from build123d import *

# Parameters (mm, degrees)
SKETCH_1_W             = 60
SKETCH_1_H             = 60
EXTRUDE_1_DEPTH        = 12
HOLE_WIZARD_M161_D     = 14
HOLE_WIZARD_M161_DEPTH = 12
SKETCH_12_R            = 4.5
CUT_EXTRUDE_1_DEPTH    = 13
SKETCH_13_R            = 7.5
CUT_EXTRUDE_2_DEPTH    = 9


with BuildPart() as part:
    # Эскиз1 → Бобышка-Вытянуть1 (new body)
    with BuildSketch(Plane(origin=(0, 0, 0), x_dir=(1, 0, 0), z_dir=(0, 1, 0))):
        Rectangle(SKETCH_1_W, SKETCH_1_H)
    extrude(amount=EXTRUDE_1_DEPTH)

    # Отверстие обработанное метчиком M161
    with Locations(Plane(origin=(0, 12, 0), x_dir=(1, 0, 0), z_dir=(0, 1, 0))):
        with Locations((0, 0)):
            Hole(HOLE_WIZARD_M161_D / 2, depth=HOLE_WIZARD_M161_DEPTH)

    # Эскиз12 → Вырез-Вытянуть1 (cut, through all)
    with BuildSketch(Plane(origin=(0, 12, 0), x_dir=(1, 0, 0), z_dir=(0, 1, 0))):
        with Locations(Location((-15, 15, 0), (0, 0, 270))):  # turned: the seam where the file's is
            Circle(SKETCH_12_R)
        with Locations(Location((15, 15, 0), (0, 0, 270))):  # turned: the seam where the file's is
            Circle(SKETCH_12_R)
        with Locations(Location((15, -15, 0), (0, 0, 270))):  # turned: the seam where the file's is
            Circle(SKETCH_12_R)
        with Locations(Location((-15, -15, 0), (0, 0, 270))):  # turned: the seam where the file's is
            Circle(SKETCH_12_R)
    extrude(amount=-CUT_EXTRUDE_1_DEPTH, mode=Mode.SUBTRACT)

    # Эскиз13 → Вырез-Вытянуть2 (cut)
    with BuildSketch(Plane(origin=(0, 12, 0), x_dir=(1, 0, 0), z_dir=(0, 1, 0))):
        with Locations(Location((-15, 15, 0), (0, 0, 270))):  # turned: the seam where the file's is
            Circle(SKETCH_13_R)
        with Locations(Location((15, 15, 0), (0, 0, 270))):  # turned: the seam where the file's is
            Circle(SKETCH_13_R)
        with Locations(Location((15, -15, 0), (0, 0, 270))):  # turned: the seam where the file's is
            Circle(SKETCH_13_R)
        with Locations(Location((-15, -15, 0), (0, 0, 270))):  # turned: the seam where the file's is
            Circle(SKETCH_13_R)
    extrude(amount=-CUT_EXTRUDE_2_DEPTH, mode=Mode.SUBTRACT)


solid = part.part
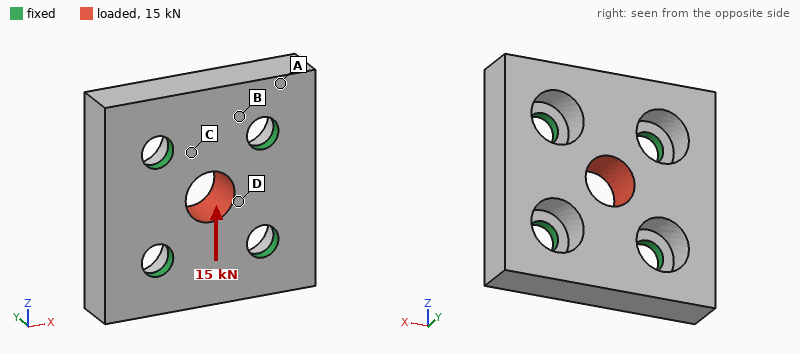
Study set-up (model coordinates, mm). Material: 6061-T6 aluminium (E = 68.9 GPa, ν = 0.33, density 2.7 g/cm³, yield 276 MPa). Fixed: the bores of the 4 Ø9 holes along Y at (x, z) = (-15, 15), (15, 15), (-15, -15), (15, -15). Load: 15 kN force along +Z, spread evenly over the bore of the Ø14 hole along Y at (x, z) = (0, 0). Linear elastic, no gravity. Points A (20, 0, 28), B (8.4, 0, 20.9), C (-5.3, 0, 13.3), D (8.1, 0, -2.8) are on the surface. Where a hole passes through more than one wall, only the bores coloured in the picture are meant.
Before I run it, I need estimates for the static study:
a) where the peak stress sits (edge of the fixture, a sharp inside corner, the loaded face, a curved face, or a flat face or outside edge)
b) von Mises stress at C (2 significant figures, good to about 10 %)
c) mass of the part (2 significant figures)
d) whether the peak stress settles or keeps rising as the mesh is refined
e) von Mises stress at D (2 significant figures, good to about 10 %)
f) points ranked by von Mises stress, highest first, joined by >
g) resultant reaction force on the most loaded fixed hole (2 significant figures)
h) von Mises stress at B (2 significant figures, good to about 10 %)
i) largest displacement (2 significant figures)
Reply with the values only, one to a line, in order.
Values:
edge of the fixture
20 MPa
92 g
keeps rising
52 MPa
D > B > C > A
4.0 kN
40 MPa
18 µm
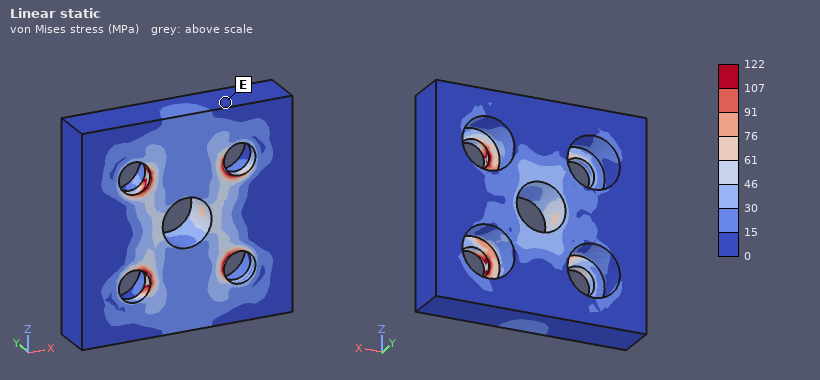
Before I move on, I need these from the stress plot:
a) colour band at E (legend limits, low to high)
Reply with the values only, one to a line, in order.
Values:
0 to 15 MPa
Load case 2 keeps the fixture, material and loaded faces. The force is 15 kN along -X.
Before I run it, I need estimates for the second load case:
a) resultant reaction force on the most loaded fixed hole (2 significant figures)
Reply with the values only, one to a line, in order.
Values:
4.0 kN
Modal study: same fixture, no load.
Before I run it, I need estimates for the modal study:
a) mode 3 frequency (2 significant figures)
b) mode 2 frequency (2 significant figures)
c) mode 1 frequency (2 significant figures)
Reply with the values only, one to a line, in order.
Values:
16 kHz
15 kHz
15 kHz
